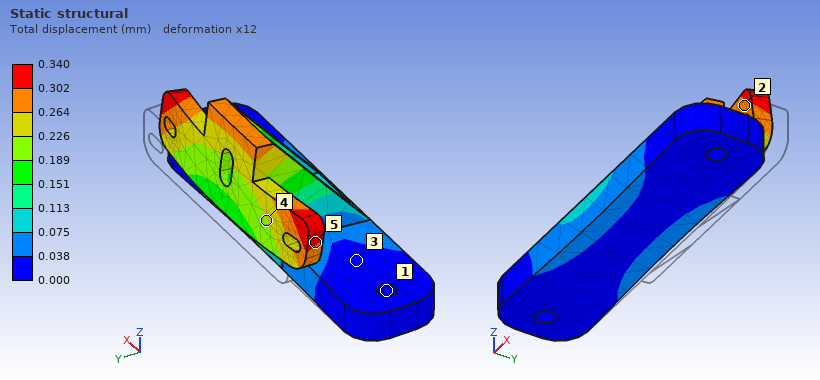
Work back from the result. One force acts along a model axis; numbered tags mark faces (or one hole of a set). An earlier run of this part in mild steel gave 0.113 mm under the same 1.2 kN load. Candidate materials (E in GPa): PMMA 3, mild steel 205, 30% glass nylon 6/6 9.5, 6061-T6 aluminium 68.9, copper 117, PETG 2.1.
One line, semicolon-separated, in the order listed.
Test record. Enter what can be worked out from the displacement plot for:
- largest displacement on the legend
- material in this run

0.340 mm; 6061-T6 aluminium
